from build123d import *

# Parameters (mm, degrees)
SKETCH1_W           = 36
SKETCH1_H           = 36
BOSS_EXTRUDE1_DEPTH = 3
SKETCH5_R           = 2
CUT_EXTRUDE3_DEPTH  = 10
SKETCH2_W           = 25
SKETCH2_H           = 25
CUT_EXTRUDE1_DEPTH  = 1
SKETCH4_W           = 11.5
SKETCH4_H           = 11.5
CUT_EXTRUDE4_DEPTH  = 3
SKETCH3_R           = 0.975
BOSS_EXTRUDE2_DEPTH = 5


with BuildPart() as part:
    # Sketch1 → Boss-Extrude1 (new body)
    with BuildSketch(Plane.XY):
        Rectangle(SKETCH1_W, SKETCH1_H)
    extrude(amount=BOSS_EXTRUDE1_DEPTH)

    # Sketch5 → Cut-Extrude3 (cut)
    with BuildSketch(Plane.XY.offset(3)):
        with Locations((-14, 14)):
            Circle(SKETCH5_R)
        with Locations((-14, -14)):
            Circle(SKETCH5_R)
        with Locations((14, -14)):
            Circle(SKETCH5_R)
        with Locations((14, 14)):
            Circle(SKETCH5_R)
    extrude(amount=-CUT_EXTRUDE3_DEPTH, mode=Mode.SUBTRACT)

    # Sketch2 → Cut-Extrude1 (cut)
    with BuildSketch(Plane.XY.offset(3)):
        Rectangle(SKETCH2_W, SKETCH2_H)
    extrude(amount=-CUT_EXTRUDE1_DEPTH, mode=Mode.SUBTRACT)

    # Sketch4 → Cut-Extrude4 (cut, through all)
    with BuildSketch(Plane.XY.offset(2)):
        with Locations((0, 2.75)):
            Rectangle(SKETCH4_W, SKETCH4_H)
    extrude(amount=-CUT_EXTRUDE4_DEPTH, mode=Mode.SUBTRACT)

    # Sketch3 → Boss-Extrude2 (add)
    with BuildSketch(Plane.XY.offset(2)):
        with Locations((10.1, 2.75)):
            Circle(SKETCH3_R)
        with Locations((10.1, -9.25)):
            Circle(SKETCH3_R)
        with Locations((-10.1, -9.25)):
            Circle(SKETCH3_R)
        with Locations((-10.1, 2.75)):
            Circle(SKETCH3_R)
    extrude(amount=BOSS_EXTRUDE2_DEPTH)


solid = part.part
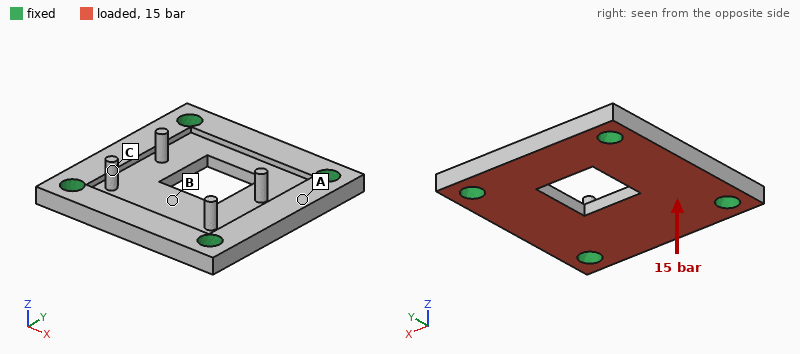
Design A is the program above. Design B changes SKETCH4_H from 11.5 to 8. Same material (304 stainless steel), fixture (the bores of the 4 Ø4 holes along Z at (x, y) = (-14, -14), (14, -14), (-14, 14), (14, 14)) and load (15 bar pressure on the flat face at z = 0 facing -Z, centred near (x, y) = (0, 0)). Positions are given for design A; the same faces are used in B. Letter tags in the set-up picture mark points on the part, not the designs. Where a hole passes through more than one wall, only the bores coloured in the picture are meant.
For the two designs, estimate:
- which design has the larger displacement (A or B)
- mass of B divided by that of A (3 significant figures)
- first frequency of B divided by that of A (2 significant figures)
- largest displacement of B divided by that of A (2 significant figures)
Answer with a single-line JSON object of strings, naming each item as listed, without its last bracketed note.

{"which design has the larger displacement": "B", "mass of B divided by that of A": "1.03", "first frequency of B divided by that of A": "0.95", "largest displacement of B divided by that of A": "1.1"}
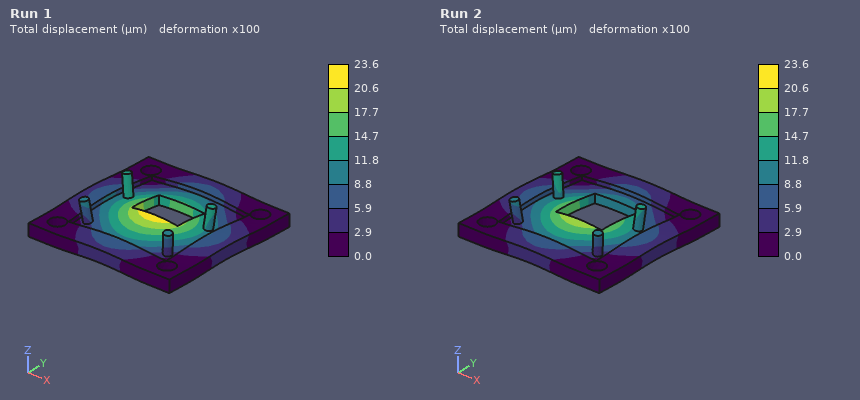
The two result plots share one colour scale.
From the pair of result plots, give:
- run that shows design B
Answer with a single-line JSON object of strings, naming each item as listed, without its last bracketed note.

{"run that shows design B": "Run 1"}
